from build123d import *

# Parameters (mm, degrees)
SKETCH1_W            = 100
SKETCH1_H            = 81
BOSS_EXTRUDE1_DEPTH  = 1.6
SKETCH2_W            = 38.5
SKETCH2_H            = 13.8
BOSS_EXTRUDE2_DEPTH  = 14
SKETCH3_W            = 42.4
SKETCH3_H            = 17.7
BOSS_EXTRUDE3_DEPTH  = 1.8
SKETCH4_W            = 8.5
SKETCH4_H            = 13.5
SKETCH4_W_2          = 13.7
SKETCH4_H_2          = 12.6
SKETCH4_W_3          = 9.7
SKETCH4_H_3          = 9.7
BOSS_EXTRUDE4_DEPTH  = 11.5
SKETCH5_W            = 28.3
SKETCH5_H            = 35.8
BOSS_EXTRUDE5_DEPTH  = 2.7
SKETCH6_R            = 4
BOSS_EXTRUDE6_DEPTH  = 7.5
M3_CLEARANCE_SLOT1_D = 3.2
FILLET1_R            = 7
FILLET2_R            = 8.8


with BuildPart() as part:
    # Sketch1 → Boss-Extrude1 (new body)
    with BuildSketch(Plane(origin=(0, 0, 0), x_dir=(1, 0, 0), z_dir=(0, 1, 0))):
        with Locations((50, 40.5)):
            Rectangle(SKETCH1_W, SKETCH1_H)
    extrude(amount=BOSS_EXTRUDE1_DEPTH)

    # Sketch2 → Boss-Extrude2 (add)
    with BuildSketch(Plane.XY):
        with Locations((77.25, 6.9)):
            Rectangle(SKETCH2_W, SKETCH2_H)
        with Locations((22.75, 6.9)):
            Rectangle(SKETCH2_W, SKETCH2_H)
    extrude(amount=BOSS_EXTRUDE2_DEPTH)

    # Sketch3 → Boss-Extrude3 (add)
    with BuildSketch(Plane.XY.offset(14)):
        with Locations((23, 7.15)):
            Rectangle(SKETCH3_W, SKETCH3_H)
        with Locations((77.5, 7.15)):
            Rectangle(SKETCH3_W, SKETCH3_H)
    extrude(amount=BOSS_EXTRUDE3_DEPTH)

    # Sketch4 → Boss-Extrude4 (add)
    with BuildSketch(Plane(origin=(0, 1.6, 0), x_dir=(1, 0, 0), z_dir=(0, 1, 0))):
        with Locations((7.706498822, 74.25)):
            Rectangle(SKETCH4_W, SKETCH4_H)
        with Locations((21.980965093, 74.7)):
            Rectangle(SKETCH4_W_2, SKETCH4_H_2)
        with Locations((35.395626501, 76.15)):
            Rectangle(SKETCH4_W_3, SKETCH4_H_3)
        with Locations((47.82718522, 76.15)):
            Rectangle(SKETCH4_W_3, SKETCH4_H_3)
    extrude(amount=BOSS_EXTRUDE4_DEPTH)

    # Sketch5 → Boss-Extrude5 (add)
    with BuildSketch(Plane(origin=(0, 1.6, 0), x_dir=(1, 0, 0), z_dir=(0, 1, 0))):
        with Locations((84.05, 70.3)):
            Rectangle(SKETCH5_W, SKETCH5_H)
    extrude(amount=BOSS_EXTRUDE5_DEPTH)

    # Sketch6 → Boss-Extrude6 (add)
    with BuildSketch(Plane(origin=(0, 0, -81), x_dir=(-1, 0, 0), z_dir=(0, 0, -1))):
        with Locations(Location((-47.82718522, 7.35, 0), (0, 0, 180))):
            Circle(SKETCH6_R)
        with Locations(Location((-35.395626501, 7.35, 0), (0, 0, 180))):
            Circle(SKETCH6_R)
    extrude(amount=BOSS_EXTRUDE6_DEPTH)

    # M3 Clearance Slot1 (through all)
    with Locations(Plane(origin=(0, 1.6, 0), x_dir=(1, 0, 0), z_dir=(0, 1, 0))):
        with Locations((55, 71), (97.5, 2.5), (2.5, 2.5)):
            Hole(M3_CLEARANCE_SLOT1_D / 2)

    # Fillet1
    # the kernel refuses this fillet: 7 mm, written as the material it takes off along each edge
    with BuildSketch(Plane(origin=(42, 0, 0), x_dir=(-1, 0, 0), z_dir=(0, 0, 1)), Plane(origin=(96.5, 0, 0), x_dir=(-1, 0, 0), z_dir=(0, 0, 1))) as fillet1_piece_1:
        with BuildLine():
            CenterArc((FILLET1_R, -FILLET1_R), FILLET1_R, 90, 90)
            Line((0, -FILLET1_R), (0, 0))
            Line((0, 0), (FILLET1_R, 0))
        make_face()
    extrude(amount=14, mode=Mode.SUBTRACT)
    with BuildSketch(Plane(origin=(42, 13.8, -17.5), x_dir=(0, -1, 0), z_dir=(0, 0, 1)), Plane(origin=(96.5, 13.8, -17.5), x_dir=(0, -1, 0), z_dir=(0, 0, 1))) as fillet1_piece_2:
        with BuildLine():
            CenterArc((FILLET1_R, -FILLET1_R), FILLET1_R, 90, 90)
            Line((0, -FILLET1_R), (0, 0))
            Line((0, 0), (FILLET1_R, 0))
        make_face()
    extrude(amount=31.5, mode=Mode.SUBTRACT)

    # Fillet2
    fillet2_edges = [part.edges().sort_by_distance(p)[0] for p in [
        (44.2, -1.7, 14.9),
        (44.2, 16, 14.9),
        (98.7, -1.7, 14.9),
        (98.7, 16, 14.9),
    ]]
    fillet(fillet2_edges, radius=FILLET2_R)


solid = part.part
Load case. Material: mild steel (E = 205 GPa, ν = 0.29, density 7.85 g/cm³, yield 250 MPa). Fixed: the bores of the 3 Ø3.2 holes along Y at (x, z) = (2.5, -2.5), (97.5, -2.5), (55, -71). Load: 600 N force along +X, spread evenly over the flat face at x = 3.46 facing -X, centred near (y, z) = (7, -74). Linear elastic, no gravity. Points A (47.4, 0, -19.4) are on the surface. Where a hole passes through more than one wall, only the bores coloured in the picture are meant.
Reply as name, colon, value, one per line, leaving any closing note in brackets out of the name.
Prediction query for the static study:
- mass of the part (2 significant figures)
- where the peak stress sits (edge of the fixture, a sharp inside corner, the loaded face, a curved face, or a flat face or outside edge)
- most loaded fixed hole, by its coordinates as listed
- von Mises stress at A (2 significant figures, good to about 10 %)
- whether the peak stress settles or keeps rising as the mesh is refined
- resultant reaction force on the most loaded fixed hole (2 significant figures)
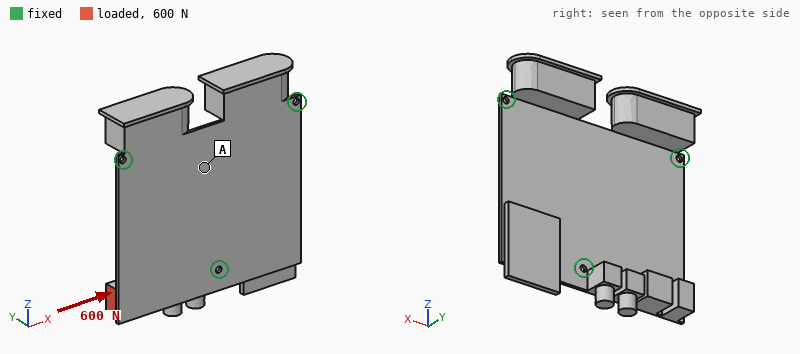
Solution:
mass of the part: 300 g
where the peak stress sits: edge of the fixture
most loaded fixed hole, by its coordinates as listed: (55, -71)
von Mises stress at A: 23 MPa
whether the peak stress settles or keeps rising as the mesh is refined: keeps rising
resultant reaction force on the most loaded fixed hole: 550 N
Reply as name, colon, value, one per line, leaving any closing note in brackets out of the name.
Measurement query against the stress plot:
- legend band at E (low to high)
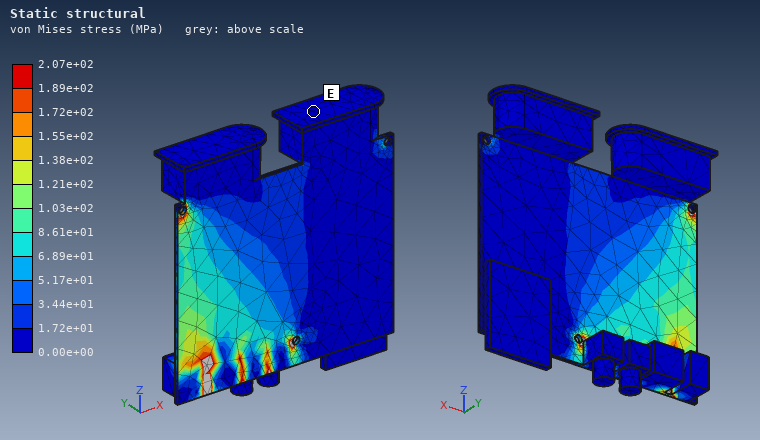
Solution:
legend band at E: 0.00e+00 to 1.72e+01 MPa
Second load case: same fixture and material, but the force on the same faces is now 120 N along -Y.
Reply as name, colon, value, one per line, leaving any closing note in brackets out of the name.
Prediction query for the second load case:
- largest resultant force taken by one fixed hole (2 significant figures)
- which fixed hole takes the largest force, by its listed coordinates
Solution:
largest resultant force taken by one fixed hole: 110 N
which fixed hole takes the largest force, by its listed coordinates: (55, -71)
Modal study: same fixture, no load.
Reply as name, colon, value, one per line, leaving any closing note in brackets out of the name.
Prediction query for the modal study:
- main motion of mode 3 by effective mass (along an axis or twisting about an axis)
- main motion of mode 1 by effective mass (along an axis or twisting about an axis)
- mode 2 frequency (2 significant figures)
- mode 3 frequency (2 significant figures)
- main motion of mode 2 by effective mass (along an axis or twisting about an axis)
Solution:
main motion of mode 3 by effective mass: along Y
main motion of mode 1 by effective mass: twisting about X
mode 2 frequency: 430 Hz
mode 3 frequency: 620 Hz
main motion of mode 2 by effective mass: along Y
